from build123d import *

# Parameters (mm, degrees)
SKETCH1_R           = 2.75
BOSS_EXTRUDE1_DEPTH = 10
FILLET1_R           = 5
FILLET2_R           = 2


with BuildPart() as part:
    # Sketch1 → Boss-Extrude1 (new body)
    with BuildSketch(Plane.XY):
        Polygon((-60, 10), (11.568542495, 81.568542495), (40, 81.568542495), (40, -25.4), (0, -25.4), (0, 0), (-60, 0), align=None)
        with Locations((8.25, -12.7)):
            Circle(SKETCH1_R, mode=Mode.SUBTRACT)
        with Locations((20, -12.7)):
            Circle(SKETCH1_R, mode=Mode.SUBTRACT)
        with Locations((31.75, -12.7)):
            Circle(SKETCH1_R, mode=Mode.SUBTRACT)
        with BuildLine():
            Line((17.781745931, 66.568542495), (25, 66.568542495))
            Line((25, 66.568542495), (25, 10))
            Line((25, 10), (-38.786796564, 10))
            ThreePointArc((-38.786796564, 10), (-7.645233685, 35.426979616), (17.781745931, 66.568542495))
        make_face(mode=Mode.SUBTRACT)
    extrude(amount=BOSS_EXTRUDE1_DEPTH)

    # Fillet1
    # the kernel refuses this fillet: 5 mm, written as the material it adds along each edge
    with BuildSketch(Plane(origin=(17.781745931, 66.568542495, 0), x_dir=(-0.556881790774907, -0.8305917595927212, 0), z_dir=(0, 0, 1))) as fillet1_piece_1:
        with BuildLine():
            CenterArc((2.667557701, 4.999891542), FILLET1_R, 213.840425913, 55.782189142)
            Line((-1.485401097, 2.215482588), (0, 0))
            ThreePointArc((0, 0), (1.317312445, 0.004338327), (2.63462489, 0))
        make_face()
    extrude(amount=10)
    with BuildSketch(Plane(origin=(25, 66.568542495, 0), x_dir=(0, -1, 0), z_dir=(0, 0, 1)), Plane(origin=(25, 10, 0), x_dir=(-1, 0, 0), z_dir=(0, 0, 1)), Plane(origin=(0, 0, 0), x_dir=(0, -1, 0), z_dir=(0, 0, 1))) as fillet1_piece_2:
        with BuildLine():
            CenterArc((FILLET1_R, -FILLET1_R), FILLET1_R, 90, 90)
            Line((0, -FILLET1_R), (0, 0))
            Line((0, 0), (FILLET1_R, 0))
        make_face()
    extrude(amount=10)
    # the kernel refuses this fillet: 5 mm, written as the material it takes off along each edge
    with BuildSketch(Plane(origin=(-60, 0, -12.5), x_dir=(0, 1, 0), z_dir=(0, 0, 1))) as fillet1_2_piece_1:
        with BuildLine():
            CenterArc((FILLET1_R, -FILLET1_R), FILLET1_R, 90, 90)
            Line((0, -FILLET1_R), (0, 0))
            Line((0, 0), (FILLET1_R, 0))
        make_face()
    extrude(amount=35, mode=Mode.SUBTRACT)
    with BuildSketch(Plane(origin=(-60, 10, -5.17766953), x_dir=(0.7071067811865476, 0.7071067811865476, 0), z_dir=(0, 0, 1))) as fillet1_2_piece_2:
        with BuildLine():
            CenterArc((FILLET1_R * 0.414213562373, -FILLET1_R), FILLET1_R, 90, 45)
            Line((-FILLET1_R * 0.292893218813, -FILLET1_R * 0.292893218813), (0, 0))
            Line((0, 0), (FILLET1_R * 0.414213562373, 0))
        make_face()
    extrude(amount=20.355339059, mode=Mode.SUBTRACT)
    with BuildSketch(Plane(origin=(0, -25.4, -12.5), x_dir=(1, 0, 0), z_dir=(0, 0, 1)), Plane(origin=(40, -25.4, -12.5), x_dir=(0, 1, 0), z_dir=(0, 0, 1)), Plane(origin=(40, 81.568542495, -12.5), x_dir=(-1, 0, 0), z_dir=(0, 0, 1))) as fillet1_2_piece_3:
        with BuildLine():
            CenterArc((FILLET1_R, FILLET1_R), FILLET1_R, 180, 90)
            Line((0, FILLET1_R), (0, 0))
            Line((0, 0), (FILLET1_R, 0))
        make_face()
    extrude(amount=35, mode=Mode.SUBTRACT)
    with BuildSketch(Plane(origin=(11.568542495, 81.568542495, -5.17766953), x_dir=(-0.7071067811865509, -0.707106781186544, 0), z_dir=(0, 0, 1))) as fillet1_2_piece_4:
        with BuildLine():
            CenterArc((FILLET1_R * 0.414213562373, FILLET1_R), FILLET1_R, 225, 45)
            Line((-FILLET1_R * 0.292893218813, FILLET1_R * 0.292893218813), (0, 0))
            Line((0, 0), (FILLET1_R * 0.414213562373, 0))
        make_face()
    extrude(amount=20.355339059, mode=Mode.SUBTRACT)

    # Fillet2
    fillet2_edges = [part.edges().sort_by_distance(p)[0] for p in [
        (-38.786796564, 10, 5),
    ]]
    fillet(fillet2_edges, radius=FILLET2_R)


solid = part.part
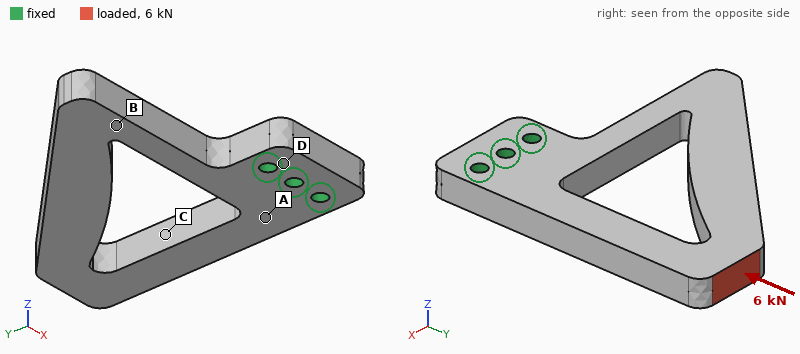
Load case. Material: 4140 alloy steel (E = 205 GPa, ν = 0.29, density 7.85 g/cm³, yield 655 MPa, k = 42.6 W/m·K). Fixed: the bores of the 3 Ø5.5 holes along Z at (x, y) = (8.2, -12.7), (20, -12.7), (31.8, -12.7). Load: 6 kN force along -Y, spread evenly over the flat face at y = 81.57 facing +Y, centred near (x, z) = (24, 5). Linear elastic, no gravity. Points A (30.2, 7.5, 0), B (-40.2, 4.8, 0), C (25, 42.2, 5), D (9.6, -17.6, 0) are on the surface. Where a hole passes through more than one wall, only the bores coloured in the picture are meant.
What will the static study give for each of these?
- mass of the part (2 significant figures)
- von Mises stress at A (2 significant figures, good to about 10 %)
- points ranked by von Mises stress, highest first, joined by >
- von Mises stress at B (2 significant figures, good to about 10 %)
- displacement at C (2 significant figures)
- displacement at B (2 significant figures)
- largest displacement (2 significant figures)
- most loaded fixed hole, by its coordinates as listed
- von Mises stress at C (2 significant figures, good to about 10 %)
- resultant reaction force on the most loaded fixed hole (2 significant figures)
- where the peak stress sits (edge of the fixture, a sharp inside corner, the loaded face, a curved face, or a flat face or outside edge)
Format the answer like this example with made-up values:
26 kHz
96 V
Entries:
370 g
36 MPa
C > A > B > D
21 MPa
13 µm
49 µm
62 µm
(31.8, -12.7)
68 MPa
3.4 kN
a curved face
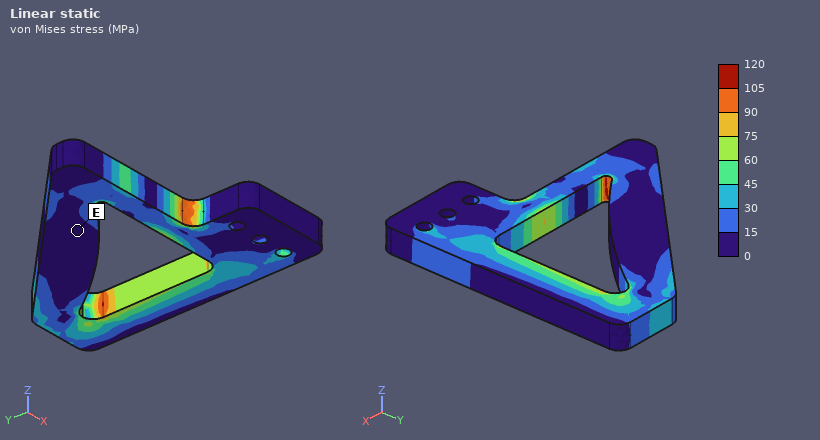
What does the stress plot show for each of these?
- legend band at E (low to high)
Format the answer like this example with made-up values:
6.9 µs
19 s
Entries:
0 to 15 MPa
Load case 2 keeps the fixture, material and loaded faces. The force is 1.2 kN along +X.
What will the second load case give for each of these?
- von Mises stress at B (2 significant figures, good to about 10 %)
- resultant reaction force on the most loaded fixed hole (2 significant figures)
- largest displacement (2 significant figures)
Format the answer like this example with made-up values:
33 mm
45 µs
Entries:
22 MPa
4.3 kN
0.12 mm
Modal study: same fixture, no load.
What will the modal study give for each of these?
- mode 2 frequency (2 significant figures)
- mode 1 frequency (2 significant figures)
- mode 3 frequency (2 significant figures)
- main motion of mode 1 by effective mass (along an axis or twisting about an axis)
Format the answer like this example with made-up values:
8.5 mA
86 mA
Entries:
1200 Hz
740 Hz
1400 Hz
along Z
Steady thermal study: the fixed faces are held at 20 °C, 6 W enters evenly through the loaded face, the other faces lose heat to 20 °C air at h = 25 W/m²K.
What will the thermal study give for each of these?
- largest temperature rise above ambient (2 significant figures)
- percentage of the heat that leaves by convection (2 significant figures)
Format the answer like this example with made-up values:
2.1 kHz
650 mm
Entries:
31 K
62 %
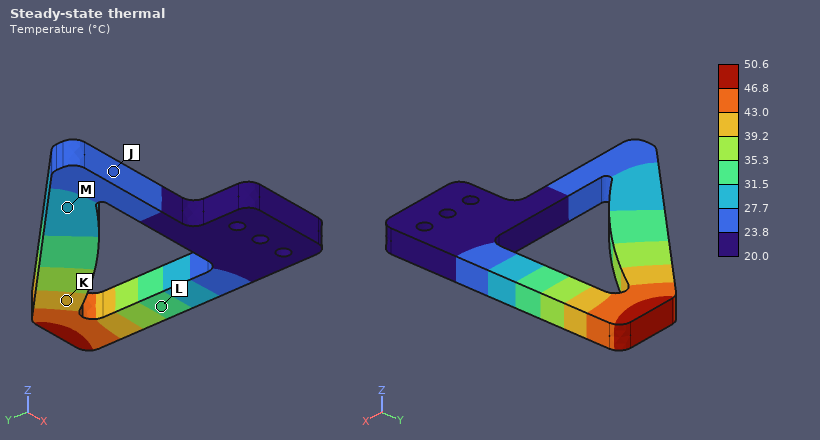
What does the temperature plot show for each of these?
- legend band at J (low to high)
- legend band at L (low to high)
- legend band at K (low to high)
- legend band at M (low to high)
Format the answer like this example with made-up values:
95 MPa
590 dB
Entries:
23.8 to 27.7 °C
31.5 to 35.3 °C
39.2 to 43.0 °C
27.7 to 31.5 °C
